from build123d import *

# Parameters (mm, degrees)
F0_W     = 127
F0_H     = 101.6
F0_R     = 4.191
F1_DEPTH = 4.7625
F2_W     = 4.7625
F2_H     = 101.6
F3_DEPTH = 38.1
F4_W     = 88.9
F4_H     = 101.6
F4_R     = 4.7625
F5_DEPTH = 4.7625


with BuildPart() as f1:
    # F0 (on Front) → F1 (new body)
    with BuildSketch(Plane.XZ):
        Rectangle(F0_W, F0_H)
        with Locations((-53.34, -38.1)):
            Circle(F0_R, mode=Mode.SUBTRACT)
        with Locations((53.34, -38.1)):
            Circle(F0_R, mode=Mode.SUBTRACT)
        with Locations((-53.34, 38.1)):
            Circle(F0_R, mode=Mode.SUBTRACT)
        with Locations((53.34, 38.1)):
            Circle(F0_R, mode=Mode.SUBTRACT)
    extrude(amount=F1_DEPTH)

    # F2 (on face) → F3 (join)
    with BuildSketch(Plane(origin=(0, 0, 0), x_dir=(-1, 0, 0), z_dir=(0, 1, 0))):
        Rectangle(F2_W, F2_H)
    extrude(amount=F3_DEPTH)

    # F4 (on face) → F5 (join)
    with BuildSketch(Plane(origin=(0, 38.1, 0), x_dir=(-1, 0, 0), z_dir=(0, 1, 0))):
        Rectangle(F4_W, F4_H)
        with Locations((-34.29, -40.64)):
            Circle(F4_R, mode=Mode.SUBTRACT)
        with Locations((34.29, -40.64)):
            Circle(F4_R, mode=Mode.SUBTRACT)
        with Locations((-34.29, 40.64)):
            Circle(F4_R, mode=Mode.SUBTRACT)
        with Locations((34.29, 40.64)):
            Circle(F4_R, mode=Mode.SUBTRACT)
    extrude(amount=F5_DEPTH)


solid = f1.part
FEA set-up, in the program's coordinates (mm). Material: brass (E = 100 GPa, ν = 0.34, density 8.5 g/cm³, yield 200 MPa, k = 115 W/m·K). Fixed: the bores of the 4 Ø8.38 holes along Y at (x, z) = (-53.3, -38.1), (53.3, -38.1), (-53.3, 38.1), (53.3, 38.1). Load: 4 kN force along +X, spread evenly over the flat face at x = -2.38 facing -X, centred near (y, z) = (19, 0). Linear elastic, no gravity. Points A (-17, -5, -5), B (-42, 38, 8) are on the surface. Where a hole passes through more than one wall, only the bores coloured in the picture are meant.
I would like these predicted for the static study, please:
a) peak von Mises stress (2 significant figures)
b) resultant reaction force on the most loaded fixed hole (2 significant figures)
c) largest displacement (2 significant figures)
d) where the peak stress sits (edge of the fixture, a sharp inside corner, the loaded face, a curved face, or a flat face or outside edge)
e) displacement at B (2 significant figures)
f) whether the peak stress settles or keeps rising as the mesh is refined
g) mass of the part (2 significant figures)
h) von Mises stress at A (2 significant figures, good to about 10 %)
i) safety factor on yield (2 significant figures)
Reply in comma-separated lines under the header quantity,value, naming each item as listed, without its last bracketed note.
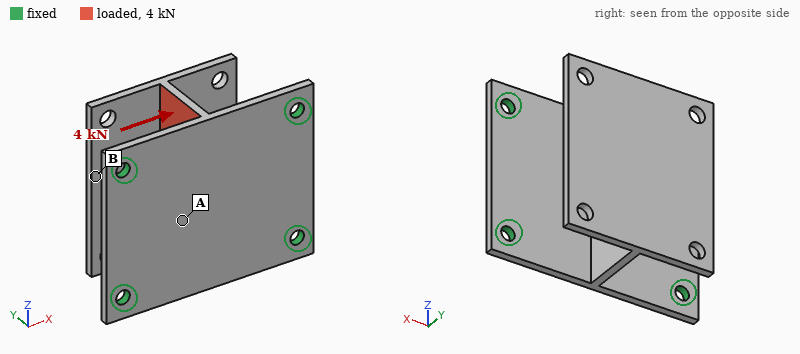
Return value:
quantity,value
peak von Mises stress,150 MPa
resultant reaction force on the most loaded fixed hole,1.2 kN
largest displacement,0.94 mm
where the peak stress sits,a flat face or outside edge
displacement at B,0.86 mm
whether the peak stress settles or keeps rising as the mesh is refined,settles
mass of the part,1.0 kg
von Mises stress at A,52 MPa
safety factor on yield,1.3
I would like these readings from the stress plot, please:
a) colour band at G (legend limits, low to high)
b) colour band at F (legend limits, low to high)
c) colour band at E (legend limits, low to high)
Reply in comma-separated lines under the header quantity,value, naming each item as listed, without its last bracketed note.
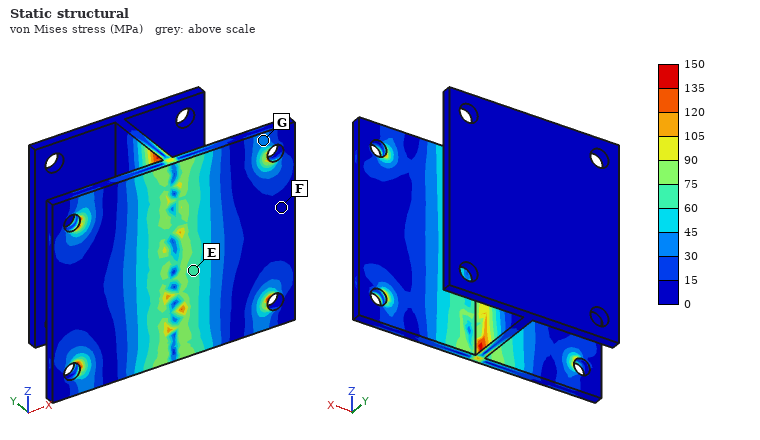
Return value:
quantity,value
colour band at G,30 to 45 MPa
colour band at F,0 to 15 MPa
colour band at E,60 to 75 MPa
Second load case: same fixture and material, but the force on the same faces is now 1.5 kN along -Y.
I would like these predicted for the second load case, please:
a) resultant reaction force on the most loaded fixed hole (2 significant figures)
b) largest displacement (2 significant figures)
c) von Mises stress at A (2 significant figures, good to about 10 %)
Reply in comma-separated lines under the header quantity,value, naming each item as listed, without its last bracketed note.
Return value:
quantity,value
resultant reaction force on the most loaded fixed hole,400 N
largest displacement,0.15 mm
von Mises stress at A,22 MPa
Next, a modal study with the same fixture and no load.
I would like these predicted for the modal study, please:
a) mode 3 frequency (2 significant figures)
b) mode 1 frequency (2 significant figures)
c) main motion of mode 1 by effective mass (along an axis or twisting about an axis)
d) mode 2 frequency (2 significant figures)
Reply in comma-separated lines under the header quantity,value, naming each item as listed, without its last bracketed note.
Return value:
quantity,value
mode 3 frequency,640 Hz
mode 1 frequency,330 Hz
main motion of mode 1 by effective mass,along X
mode 2 frequency,630 Hz
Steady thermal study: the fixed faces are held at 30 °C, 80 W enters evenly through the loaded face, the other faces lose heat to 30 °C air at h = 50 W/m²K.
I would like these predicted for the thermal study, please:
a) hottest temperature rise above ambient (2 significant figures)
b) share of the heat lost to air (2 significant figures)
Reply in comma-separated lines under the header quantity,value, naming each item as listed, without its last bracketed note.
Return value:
quantity,value
hottest temperature rise above ambient,33 K
share of the heat lost to air,57 %
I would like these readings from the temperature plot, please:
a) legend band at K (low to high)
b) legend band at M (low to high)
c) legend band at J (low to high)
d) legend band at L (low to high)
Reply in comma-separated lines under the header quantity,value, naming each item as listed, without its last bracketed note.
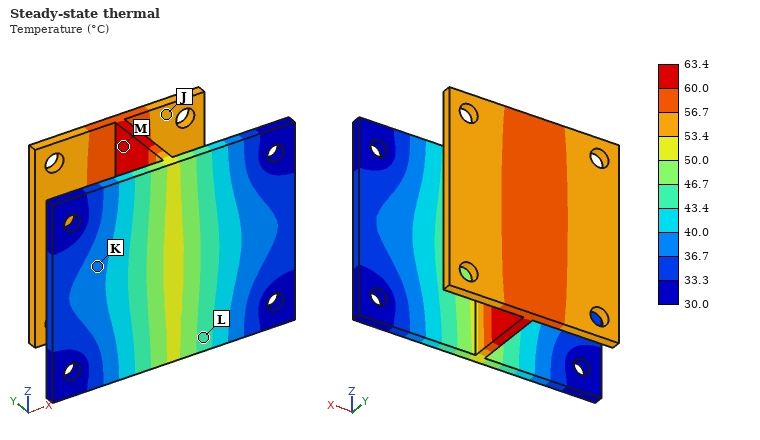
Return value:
quantity,value
legend band at K,36.7 to 40.0 °C
legend band at M,60.0 to 63.4 °C
legend band at J,53.4 to 56.7 °C
legend band at L,43.4 to 46.7 °C
